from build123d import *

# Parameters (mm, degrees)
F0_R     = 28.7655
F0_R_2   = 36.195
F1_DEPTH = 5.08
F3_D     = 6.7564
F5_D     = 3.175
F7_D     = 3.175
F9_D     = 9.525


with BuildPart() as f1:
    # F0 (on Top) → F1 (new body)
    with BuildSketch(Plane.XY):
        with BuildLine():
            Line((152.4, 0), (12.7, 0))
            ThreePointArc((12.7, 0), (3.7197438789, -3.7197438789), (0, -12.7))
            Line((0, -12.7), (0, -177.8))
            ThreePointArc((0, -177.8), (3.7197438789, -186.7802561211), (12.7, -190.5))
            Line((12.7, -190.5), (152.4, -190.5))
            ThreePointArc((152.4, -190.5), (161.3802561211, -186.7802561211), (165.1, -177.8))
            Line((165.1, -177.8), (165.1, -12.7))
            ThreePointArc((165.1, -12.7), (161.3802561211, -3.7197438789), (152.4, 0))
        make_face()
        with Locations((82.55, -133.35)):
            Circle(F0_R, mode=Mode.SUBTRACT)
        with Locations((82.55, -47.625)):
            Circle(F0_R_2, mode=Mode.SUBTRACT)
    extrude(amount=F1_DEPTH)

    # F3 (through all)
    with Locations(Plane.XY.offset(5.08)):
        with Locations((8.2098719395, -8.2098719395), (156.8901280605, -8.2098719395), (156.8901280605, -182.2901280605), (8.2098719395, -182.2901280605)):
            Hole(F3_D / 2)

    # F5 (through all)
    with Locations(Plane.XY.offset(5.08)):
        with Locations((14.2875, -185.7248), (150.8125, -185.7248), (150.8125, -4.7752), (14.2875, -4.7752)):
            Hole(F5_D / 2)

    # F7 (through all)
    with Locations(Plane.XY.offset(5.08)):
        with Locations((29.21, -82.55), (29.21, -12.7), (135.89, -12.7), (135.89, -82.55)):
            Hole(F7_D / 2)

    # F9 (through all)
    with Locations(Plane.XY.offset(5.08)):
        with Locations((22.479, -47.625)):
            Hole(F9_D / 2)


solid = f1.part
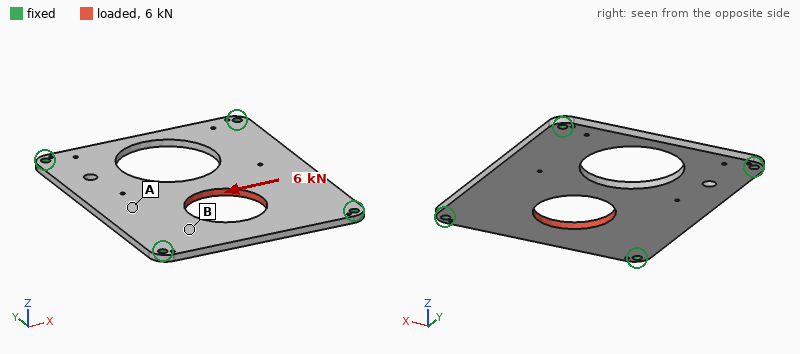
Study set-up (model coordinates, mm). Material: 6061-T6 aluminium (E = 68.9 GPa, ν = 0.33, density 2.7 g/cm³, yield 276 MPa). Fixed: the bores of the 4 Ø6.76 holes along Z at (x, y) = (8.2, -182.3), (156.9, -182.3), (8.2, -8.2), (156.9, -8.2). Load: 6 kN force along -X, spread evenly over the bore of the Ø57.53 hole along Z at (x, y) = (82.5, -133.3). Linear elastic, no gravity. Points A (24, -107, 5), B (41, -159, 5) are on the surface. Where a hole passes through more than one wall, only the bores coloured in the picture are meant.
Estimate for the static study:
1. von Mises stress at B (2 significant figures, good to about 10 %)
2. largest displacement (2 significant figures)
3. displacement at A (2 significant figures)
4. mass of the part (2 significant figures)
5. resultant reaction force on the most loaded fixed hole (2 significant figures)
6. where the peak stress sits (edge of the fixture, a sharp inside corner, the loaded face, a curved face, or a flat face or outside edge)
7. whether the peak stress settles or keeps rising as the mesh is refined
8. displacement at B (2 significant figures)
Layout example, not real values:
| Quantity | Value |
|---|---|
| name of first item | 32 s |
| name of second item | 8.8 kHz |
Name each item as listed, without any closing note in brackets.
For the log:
| Quantity | Value |
|---|---|
| von Mises stress at B | 9.6 MPa |
| largest displacement | 25 µm |
| displacement at A | 24 µm |
| mass of the part | 330 g |
| resultant reaction force on the most loaded fixed hole | 2.5 kN |
| where the peak stress sits | edge of the fixture |
| whether the peak stress settles or keeps rising as the mesh is refined | keeps rising |
| displacement at B | 13 µm |
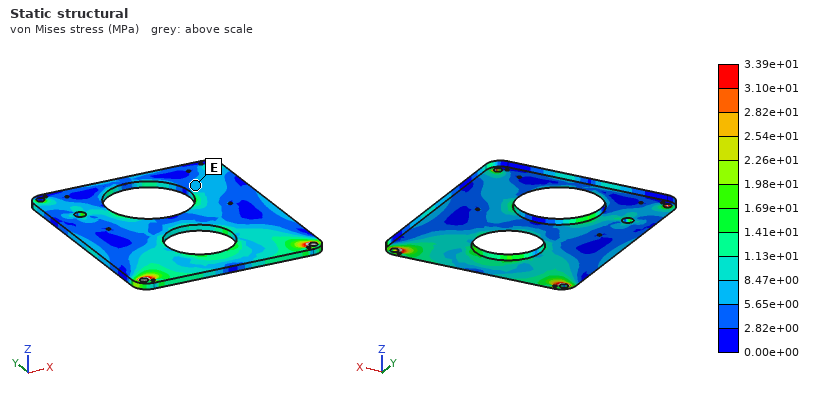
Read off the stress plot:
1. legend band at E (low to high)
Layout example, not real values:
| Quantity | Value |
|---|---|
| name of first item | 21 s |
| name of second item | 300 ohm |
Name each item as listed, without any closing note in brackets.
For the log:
| Quantity | Value |
|---|---|
| legend band at E | 5.65e+00 to 8.47e+00 MPa |
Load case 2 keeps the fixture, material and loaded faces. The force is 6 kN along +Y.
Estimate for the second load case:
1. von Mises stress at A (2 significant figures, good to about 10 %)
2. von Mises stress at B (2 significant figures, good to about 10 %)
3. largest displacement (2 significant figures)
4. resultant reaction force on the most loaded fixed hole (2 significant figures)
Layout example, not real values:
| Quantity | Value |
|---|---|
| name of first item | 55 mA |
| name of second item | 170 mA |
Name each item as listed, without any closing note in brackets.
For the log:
| Quantity | Value |
|---|---|
| von Mises stress at A | 5.9 MPa |
| von Mises stress at B | 7.7 MPa |
| largest displacement | 26 µm |
| resultant reaction force on the most loaded fixed hole | 1.9 kN |
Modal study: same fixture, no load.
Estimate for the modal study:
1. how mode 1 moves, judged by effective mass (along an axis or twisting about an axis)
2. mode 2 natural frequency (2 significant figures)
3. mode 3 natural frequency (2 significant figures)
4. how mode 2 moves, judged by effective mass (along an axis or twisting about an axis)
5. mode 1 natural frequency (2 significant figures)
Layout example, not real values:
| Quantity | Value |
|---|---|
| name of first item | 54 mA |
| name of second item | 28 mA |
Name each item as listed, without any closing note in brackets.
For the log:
| Quantity | Value |
|---|---|
| how mode 1 moves, judged by effective mass | along Z |
| mode 2 natural frequency | 950 Hz |
| mode 3 natural frequency | 1200 Hz |
| how mode 2 moves, judged by effective mass | twisting about Y |
| mode 1 natural frequency | 620 Hz |
